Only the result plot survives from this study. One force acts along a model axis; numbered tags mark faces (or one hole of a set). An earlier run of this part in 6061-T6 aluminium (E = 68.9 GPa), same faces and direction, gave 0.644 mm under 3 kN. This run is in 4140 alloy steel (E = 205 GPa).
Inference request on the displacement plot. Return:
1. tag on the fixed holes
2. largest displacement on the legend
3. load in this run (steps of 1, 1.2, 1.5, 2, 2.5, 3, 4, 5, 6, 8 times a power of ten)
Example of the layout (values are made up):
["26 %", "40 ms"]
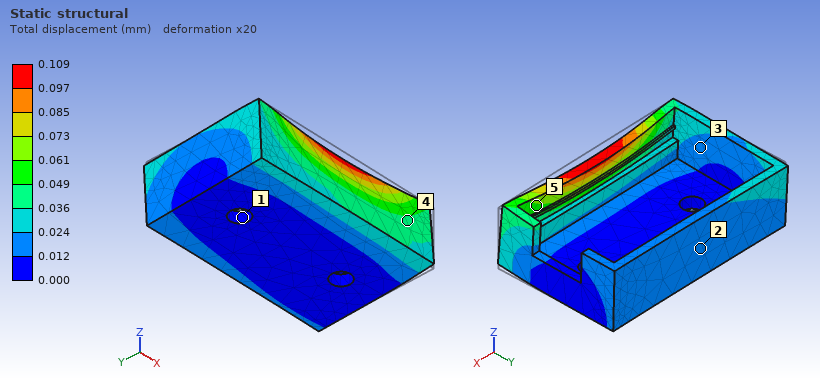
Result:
["1", "0.109 mm", "1.5 kN"]
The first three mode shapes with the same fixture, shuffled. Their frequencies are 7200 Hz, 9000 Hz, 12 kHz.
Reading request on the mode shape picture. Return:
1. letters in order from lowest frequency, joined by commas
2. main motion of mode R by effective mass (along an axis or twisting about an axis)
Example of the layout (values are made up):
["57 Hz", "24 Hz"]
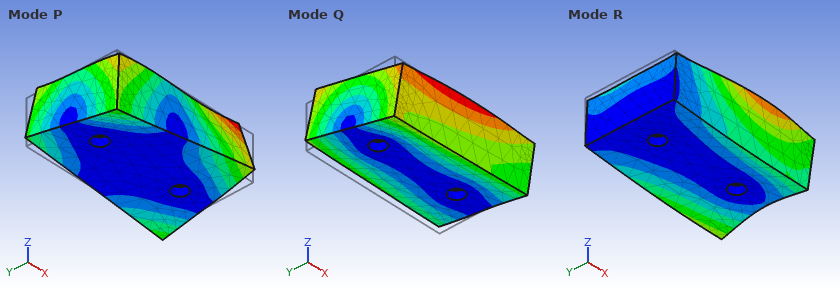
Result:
["Q, P, R", "along Z"]
